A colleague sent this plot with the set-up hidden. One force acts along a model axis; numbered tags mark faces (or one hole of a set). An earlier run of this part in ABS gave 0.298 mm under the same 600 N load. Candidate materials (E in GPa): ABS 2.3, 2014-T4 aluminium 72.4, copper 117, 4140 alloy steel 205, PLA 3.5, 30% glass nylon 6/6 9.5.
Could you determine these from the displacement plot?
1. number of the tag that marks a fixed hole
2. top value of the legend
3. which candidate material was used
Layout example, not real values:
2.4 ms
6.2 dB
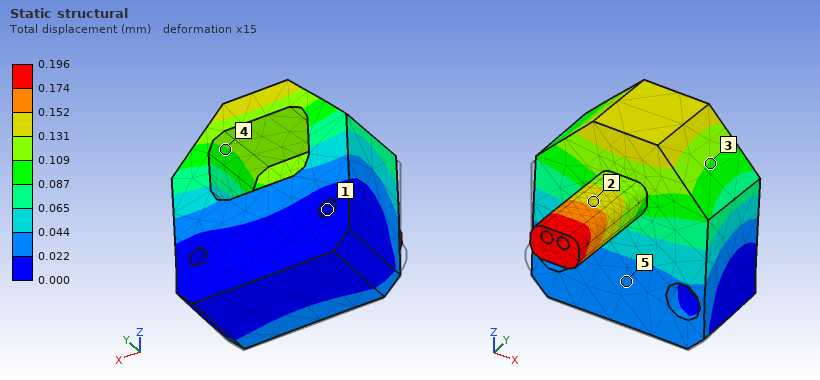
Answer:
1
0.196 mm
PLA
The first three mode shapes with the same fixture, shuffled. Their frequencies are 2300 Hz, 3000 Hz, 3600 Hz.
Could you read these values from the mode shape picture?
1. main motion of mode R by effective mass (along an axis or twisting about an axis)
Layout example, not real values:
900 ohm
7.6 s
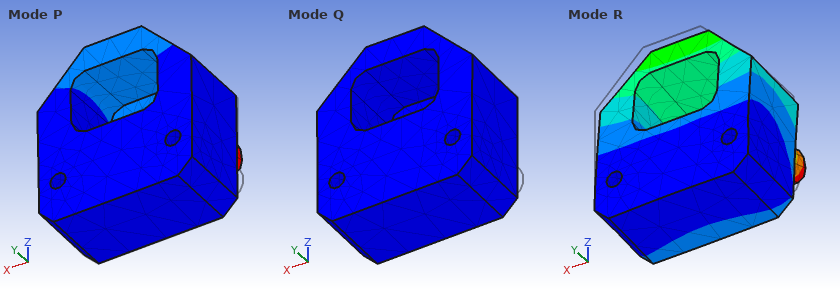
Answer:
along Y
